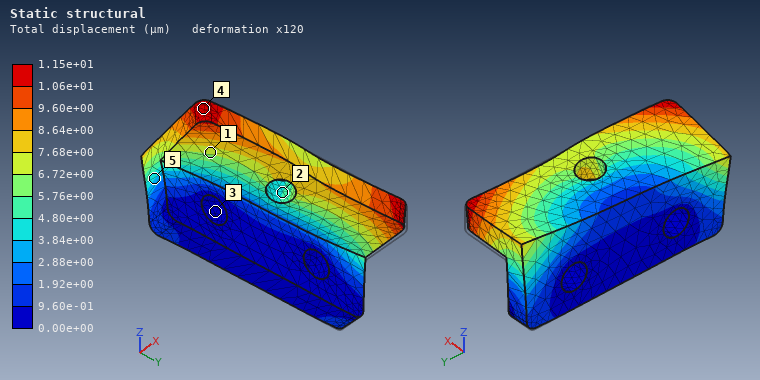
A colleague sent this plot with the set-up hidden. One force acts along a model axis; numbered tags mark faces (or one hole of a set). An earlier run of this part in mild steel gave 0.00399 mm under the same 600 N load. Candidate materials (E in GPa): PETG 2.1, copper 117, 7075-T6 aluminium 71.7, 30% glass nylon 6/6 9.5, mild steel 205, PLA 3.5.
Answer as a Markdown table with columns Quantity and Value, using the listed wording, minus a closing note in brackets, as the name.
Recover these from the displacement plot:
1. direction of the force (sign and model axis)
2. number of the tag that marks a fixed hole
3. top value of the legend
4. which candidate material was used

| Quantity | Value |
|---|---|
| direction of the force | -Y |
| number of the tag that marks a fixed hole | 3 |
| top value of the legend | 1.15e+01 µm |
| which candidate material was used | 7075-T6 aluminium |
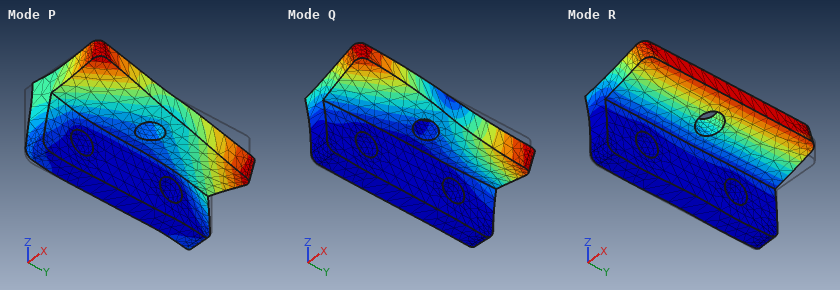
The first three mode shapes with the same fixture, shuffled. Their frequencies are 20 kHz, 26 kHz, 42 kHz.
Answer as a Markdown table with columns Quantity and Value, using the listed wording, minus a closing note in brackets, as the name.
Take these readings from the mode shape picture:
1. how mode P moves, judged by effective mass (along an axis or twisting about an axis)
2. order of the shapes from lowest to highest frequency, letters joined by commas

| Quantity | Value |
|---|---|
| how mode P moves, judged by effective mass | along Y |
| order of the shapes from lowest to highest frequency, letters joined by commas | R, Q, P |
